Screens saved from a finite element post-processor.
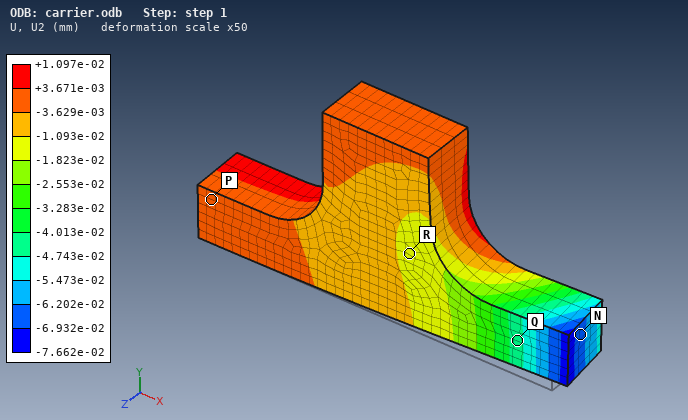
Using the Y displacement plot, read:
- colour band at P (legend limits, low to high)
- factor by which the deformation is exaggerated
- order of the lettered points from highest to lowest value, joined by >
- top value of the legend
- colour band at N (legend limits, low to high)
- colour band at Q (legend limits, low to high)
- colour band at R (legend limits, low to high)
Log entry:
-3.629e-03 to +3.671e-03 mm
50
P > R > Q > N
+1.097e-02 mm
-6.932e-02 to -6.202e-02 mm
-4.743e-02 to -4.013e-02 mm
-1.823e-02 to -1.093e-02 mm
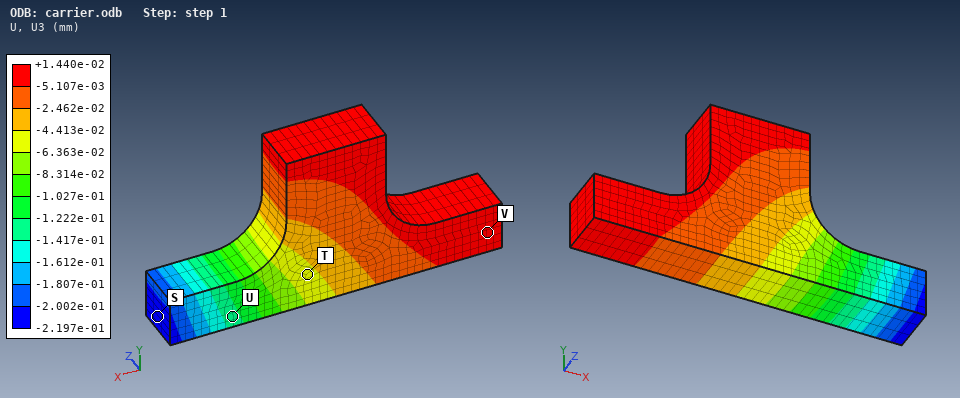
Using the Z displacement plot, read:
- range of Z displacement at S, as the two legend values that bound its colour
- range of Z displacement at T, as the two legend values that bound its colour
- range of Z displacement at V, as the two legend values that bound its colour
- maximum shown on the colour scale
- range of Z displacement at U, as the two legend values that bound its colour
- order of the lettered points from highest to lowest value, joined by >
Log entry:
-2.197e-01 to -2.002e-01 mm
-6.363e-02 to -4.413e-02 mm
-5.107e-03 to +1.440e-02 mm
+1.440e-02 mm
-1.417e-01 to -1.222e-01 mm
V > T > U > S
